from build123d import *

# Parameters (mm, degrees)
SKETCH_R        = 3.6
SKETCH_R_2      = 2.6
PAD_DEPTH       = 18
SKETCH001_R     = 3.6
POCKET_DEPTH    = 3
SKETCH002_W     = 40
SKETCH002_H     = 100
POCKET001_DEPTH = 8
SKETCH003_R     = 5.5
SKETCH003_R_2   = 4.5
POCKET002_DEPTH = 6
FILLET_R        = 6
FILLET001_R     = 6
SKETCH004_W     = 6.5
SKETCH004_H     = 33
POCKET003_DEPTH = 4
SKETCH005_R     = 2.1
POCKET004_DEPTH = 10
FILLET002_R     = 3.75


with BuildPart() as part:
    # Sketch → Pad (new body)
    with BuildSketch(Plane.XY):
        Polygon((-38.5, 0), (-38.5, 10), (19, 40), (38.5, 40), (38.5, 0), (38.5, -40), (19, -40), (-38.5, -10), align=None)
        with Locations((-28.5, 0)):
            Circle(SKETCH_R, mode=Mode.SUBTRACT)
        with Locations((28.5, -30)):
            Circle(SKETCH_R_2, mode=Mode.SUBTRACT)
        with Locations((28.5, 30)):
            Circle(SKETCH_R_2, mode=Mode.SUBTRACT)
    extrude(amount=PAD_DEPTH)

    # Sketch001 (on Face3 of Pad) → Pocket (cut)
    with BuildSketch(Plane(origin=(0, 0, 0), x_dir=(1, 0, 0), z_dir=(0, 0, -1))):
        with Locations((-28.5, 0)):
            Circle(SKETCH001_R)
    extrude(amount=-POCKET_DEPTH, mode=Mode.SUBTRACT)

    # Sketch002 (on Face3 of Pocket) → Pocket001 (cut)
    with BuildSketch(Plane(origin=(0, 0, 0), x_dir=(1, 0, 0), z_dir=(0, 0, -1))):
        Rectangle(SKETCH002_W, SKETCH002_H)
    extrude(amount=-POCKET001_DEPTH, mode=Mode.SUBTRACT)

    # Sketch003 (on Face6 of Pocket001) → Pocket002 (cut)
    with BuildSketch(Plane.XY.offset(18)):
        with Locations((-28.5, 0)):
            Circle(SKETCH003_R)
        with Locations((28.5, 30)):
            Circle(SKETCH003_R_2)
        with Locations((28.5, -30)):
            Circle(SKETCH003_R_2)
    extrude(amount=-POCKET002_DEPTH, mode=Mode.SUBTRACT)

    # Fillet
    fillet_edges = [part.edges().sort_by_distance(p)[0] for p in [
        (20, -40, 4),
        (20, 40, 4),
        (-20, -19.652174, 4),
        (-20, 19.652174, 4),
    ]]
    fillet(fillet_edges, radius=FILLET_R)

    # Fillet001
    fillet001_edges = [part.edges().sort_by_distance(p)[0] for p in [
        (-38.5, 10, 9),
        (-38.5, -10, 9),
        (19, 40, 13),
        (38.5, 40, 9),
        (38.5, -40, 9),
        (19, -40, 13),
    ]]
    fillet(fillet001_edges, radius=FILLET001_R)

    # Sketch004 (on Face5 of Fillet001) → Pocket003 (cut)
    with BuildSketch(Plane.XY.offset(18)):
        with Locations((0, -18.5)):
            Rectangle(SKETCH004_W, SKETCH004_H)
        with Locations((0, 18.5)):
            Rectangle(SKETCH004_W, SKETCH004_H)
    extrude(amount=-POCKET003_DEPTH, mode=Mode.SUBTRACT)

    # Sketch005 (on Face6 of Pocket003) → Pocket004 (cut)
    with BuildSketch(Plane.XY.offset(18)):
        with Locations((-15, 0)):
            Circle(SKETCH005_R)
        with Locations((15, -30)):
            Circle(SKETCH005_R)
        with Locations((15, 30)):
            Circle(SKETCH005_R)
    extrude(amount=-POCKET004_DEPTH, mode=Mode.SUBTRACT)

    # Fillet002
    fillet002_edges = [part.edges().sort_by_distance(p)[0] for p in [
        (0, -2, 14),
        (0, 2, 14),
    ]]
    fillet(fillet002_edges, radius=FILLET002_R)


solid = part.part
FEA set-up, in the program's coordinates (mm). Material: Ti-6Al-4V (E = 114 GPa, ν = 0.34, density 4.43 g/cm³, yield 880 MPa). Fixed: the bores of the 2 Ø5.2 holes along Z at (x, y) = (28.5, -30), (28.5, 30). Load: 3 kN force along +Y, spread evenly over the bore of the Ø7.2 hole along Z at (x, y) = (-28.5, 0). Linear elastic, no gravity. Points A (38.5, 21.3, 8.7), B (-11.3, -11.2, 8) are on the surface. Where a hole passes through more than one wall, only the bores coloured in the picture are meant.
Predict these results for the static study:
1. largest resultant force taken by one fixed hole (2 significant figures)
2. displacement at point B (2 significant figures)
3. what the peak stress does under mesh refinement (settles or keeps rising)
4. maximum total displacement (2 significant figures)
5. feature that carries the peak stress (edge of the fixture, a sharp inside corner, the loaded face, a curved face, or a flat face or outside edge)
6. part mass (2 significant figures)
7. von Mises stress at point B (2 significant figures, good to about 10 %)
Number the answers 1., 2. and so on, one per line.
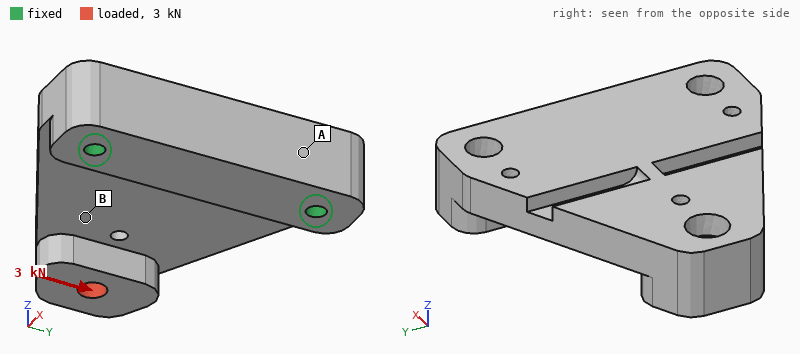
1. 3.1 kN
2. 18 µm
3. keeps rising
4. 42 µm
5. edge of the fixture
6. 250 g
7. 37 MPa
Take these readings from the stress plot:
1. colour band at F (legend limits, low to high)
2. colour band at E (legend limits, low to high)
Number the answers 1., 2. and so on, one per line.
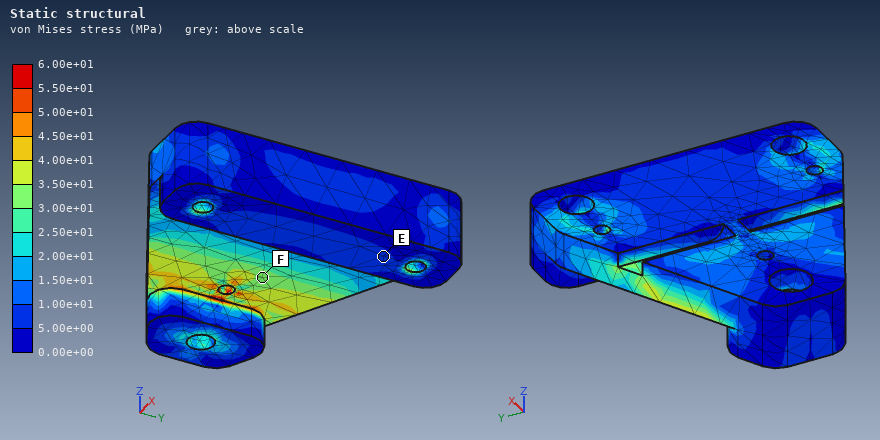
1. 3.00e+01 to 3.50e+01 MPa
2. 5.00e+00 to 1.00e+01 MPa
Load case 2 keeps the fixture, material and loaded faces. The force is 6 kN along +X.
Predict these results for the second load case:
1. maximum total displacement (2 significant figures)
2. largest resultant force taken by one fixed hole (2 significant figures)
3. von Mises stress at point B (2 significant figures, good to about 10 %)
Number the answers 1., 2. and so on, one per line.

1. 0.22 mm
2. 3.1 kN
3. 71 MPa
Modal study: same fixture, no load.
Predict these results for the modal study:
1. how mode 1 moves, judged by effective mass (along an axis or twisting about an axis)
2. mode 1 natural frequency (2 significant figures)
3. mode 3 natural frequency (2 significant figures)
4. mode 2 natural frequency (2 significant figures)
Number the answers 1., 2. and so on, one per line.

1. along Z
2. 1800 Hz
3. 7600 Hz
4. 6500 Hz
